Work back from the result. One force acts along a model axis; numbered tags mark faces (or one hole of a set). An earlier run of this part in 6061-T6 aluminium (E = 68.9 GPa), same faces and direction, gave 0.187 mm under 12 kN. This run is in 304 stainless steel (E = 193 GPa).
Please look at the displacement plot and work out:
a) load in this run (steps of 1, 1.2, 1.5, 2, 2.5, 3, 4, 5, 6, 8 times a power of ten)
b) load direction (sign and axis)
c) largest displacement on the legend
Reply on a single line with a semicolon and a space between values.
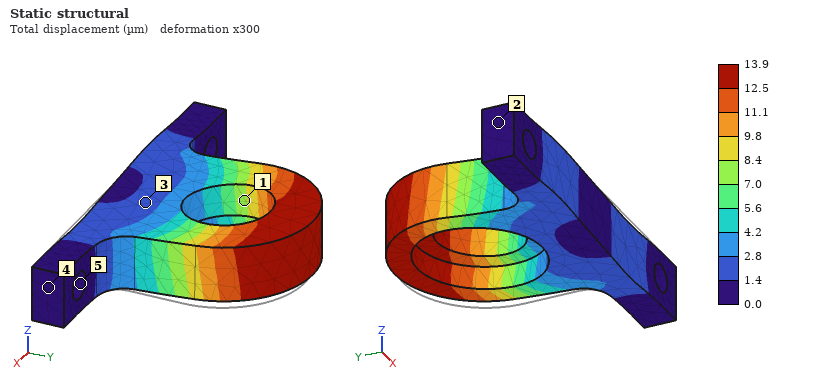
2.5 kN; -X; 13.9 µm
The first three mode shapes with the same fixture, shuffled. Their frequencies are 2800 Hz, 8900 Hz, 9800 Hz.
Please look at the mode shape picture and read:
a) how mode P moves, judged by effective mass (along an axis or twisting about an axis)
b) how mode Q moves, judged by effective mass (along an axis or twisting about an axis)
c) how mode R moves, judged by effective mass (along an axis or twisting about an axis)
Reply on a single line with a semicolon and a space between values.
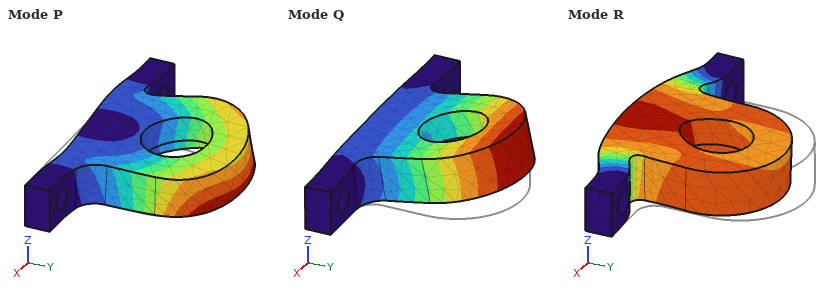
along X; along Z; along Y
